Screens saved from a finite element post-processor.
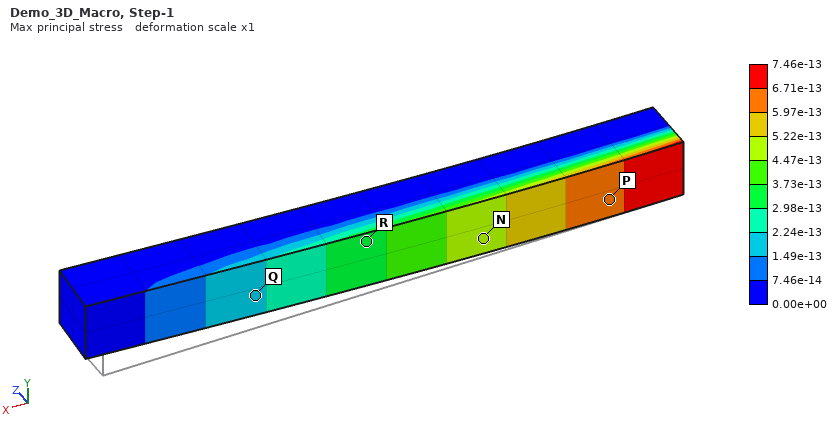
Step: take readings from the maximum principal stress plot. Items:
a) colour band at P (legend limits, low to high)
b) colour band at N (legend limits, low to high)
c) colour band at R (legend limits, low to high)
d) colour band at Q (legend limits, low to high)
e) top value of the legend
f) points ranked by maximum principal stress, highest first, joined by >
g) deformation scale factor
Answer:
5.97e-13 to 6.71e-13
4.47e-13 to 5.22e-13
2.98e-13 to 3.73e-13
1.49e-13 to 2.24e-13
7.46e-13
P > N > R > Q
1
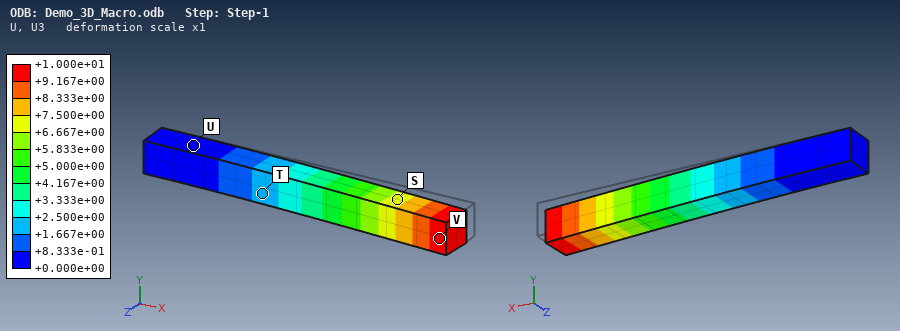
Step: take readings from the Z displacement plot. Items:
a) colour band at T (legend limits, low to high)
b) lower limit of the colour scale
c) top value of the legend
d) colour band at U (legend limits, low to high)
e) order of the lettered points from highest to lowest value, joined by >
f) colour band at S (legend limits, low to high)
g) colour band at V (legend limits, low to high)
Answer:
+1.667e+00 to +2.500e+00
+0.000e+00
+1.000e+01
+0.000e+00 to +8.333e-01
V > S > T > U
+6.667e+00 to +7.500e+00
+9.167e+00 to +1.000e+01
